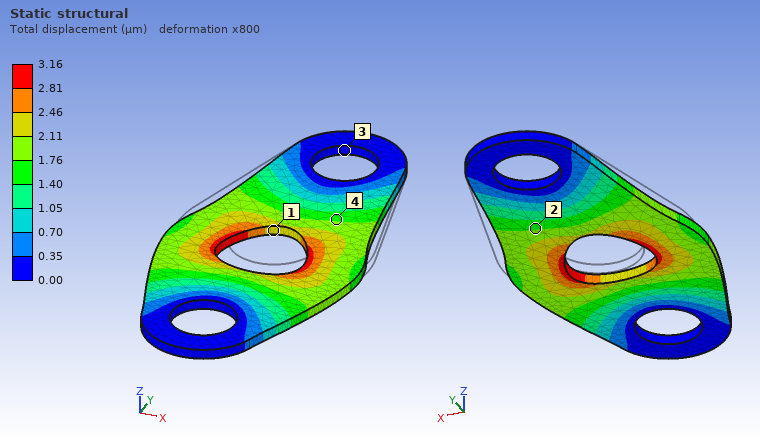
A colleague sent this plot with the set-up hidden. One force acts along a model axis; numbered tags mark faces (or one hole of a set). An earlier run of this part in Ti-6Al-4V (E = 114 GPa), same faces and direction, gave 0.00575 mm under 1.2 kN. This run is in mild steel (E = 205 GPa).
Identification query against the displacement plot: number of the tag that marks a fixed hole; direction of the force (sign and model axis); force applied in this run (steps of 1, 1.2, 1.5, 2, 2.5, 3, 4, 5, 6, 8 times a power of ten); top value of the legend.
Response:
3
-Y
1.2 kN
3.16 µm
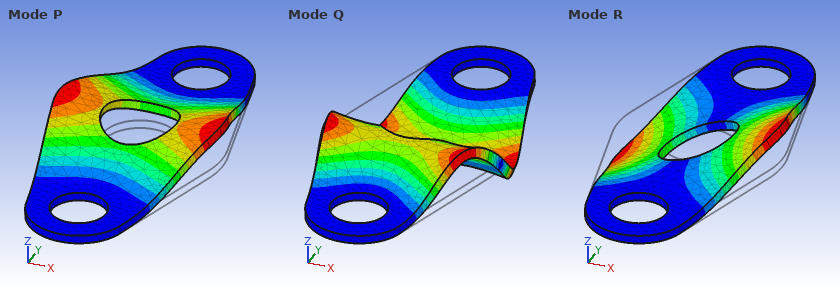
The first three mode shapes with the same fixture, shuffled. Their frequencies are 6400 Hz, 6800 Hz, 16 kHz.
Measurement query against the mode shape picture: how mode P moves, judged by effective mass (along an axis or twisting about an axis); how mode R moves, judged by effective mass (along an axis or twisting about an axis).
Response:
along Z
twisting about Y
